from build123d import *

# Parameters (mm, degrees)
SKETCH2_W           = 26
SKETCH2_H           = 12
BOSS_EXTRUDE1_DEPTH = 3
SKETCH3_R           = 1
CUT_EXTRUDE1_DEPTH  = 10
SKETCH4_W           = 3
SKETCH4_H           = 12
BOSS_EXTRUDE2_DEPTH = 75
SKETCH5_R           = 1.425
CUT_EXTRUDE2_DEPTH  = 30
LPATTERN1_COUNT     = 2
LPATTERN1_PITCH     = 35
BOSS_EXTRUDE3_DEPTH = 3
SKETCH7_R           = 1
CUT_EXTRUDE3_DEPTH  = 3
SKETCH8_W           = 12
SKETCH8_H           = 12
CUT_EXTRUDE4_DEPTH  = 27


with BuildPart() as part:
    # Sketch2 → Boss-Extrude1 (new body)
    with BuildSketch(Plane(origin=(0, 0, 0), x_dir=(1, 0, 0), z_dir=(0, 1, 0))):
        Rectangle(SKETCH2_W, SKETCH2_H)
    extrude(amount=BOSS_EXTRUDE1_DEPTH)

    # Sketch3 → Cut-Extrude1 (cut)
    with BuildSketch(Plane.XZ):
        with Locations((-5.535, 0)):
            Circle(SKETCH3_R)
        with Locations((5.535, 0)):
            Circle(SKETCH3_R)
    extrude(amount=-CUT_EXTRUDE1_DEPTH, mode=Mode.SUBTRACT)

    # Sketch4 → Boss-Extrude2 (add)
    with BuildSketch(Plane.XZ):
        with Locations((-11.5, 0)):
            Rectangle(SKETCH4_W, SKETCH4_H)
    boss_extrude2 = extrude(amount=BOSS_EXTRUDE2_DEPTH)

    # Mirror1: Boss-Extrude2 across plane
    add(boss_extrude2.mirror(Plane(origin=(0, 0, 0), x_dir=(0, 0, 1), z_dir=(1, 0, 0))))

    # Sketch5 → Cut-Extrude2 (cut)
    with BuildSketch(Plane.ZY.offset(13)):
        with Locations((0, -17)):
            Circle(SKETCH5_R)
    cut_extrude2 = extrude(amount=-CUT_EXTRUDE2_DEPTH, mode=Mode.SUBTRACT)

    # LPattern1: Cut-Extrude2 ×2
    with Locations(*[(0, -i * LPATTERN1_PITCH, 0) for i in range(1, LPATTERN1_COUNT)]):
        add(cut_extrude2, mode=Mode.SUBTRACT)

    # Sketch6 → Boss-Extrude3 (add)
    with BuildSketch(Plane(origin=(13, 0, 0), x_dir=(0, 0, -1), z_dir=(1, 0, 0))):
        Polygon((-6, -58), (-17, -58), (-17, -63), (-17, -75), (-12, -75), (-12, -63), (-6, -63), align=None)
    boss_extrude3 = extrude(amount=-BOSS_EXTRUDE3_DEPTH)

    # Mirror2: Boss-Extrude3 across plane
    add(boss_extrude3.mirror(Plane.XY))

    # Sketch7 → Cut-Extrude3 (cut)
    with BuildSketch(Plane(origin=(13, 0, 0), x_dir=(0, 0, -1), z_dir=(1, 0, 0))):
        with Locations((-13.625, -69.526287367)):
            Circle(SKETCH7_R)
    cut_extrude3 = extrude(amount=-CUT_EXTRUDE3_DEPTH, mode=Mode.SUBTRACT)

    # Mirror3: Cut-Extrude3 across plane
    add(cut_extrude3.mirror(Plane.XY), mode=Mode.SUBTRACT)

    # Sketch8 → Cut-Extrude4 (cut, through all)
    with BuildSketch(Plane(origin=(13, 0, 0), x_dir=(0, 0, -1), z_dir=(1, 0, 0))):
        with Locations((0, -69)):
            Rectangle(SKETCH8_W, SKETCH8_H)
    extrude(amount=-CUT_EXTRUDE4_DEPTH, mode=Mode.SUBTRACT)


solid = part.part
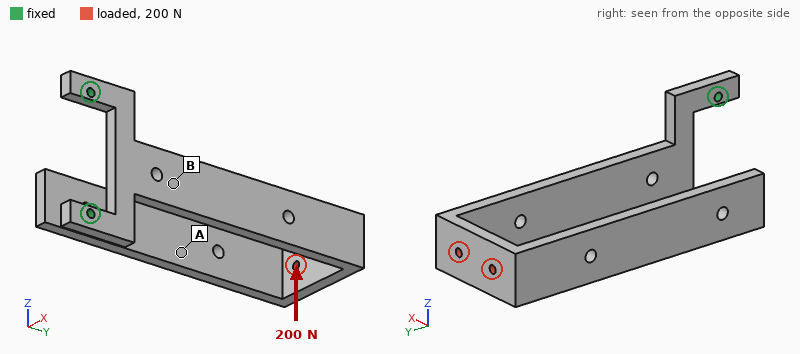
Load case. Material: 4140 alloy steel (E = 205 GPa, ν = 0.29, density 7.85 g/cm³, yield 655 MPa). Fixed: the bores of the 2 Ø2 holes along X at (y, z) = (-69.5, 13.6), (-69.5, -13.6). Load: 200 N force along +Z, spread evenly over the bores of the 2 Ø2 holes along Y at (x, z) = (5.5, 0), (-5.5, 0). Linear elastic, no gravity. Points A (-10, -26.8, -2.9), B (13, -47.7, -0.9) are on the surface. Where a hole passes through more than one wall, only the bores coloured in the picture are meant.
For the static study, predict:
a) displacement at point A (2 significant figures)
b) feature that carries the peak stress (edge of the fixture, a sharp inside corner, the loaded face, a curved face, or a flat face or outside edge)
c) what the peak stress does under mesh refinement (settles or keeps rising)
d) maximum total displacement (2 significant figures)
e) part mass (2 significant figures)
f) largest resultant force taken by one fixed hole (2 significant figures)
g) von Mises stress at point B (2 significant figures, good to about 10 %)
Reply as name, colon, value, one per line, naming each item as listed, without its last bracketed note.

displacement at point A: 0.57 mm
feature that carries the peak stress: a sharp inside corner
what the peak stress does under mesh refinement: keeps rising
maximum total displacement: 0.81 mm
part mass: 47 g
largest resultant force taken by one fixed hole: 540 N
von Mises stress at point B: 120 MPa
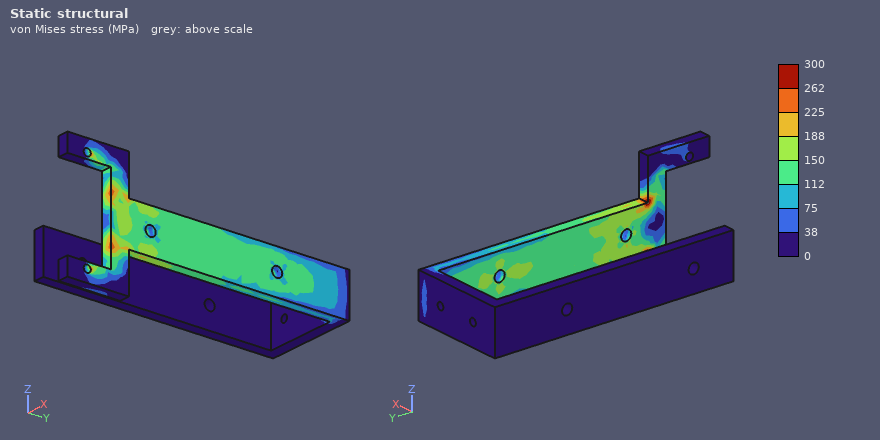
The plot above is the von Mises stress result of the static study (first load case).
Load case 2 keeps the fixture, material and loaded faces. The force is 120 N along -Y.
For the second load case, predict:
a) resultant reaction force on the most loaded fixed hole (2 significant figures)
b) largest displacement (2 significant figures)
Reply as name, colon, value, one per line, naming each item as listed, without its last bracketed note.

resultant reaction force on the most loaded fixed hole: 70 N
largest displacement: 0.99 mm
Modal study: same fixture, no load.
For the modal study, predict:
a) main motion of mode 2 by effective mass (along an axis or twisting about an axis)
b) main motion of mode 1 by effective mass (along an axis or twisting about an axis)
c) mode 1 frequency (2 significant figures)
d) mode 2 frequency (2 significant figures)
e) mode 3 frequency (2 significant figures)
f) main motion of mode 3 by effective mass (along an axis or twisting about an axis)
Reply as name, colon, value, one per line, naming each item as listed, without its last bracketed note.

main motion of mode 2 by effective mass: along X
main motion of mode 1 by effective mass: along X
mode 1 frequency: 210 Hz
mode 2 frequency: 300 Hz
mode 3 frequency: 390 Hz
main motion of mode 3 by effective mass: along Z
